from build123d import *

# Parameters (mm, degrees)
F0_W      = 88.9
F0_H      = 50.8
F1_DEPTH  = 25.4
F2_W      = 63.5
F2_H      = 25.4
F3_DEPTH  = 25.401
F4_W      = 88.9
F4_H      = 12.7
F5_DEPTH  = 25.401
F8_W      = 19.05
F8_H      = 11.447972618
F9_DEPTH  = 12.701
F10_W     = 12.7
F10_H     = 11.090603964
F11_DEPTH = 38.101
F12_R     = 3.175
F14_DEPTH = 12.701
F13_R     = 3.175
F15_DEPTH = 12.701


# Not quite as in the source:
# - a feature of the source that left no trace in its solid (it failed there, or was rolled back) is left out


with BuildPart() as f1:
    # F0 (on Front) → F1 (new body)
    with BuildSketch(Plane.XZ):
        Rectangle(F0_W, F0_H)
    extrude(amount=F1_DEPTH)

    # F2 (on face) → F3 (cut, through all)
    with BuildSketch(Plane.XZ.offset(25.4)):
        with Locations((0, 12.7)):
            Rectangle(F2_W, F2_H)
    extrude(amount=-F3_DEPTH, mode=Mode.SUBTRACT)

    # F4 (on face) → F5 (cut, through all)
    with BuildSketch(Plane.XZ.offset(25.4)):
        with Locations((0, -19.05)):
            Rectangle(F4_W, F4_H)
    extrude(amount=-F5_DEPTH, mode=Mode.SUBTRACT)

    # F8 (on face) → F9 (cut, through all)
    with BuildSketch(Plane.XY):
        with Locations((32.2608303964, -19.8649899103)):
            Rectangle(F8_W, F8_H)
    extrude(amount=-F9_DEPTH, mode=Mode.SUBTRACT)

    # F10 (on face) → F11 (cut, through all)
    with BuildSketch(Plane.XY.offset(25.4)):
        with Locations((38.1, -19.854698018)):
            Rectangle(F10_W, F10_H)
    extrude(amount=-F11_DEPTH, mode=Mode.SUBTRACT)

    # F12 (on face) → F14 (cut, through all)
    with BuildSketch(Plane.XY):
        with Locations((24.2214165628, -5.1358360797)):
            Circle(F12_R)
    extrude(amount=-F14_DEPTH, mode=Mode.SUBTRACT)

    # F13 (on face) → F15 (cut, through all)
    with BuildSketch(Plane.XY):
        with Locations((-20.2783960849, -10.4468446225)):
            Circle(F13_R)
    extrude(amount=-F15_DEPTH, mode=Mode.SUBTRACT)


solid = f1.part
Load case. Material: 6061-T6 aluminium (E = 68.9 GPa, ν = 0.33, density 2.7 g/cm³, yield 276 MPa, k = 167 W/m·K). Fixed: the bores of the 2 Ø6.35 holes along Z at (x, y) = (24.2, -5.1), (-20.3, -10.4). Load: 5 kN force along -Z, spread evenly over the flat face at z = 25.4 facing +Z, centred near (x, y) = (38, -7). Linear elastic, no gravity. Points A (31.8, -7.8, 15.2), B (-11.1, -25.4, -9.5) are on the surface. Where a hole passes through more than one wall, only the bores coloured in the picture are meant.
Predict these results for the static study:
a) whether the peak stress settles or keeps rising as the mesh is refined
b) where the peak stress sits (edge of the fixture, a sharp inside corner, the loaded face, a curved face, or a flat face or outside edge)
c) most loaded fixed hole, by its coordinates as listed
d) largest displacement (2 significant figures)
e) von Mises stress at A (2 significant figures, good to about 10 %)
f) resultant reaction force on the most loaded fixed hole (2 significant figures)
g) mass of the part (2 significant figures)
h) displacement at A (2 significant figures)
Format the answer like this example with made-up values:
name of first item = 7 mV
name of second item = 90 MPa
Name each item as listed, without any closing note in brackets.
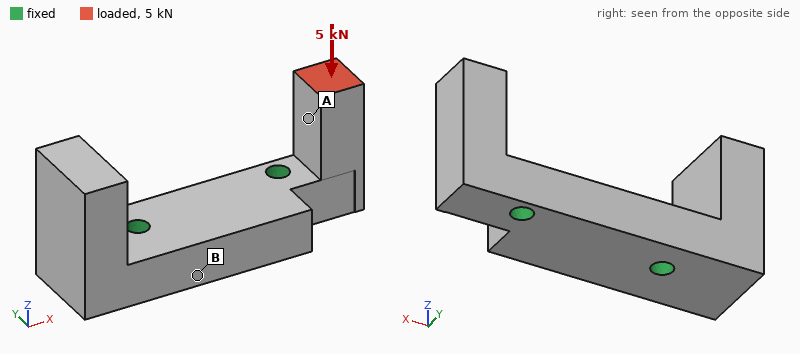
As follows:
whether the peak stress settles or keeps rising as the mesh is refined = keeps rising
where the peak stress sits = edge of the fixture
most loaded fixed hole, by its coordinates as listed = (24.2, -5.1)
largest displacement = 0.11 mm
von Mises stress at A = 28 MPa
resultant reaction force on the most loaded fixed hole = 5.1 kN
mass of the part = 100 g
displacement at A = 0.064 mm
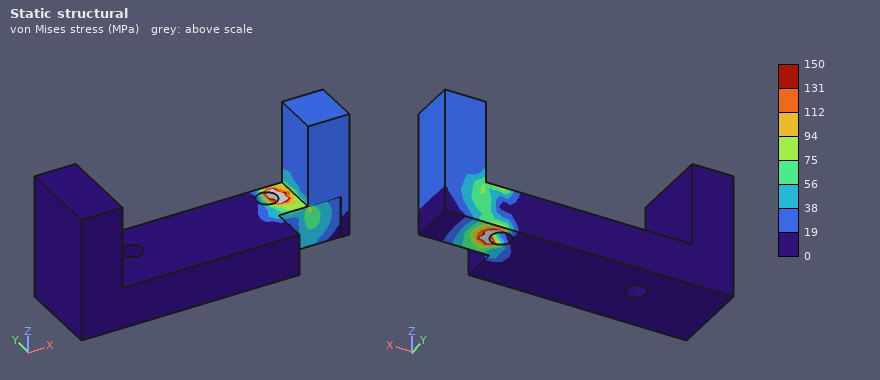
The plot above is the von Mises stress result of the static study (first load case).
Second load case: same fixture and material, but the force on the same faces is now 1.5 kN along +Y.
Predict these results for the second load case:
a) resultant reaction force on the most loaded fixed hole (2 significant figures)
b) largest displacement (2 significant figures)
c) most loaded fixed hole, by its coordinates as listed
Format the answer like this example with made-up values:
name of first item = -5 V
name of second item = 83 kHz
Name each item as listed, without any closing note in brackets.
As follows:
resultant reaction force on the most loaded fixed hole = 1.6 kN
largest displacement = 0.20 mm
most loaded fixed hole, by its coordinates as listed = (24.2, -5.1)
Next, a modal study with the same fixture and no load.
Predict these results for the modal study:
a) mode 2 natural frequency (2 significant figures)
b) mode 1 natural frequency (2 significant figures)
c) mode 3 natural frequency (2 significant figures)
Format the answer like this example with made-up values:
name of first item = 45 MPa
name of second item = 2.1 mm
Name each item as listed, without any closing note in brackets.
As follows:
mode 2 natural frequency = 6100 Hz
mode 1 natural frequency = 5300 Hz
mode 3 natural frequency = 6200 Hz
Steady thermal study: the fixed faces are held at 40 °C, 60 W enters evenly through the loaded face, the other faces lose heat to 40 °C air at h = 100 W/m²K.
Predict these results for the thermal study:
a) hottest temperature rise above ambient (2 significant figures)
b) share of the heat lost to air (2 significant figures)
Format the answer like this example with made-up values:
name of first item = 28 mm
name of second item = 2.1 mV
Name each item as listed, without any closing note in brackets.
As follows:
hottest temperature rise above ambient = 70 K
share of the heat lost to air = 13 %
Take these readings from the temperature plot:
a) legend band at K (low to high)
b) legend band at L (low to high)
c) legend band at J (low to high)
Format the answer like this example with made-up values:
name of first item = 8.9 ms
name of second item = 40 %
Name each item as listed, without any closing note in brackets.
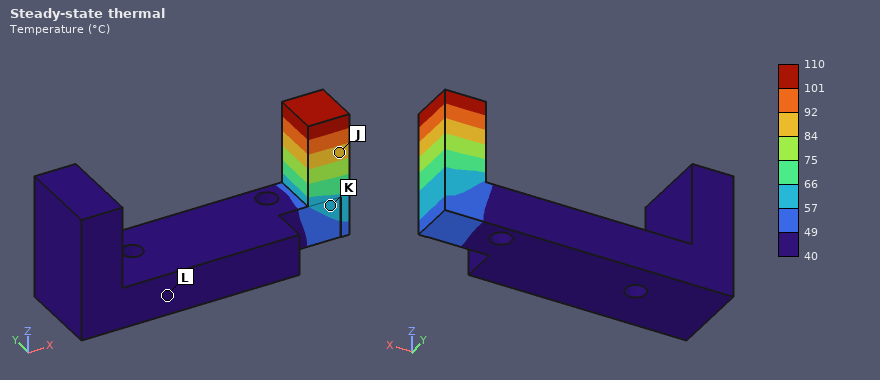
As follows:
legend band at K = 57 to 66 °C
legend band at L = 40 to 49 °C
legend band at J = 84 to 92 °C
